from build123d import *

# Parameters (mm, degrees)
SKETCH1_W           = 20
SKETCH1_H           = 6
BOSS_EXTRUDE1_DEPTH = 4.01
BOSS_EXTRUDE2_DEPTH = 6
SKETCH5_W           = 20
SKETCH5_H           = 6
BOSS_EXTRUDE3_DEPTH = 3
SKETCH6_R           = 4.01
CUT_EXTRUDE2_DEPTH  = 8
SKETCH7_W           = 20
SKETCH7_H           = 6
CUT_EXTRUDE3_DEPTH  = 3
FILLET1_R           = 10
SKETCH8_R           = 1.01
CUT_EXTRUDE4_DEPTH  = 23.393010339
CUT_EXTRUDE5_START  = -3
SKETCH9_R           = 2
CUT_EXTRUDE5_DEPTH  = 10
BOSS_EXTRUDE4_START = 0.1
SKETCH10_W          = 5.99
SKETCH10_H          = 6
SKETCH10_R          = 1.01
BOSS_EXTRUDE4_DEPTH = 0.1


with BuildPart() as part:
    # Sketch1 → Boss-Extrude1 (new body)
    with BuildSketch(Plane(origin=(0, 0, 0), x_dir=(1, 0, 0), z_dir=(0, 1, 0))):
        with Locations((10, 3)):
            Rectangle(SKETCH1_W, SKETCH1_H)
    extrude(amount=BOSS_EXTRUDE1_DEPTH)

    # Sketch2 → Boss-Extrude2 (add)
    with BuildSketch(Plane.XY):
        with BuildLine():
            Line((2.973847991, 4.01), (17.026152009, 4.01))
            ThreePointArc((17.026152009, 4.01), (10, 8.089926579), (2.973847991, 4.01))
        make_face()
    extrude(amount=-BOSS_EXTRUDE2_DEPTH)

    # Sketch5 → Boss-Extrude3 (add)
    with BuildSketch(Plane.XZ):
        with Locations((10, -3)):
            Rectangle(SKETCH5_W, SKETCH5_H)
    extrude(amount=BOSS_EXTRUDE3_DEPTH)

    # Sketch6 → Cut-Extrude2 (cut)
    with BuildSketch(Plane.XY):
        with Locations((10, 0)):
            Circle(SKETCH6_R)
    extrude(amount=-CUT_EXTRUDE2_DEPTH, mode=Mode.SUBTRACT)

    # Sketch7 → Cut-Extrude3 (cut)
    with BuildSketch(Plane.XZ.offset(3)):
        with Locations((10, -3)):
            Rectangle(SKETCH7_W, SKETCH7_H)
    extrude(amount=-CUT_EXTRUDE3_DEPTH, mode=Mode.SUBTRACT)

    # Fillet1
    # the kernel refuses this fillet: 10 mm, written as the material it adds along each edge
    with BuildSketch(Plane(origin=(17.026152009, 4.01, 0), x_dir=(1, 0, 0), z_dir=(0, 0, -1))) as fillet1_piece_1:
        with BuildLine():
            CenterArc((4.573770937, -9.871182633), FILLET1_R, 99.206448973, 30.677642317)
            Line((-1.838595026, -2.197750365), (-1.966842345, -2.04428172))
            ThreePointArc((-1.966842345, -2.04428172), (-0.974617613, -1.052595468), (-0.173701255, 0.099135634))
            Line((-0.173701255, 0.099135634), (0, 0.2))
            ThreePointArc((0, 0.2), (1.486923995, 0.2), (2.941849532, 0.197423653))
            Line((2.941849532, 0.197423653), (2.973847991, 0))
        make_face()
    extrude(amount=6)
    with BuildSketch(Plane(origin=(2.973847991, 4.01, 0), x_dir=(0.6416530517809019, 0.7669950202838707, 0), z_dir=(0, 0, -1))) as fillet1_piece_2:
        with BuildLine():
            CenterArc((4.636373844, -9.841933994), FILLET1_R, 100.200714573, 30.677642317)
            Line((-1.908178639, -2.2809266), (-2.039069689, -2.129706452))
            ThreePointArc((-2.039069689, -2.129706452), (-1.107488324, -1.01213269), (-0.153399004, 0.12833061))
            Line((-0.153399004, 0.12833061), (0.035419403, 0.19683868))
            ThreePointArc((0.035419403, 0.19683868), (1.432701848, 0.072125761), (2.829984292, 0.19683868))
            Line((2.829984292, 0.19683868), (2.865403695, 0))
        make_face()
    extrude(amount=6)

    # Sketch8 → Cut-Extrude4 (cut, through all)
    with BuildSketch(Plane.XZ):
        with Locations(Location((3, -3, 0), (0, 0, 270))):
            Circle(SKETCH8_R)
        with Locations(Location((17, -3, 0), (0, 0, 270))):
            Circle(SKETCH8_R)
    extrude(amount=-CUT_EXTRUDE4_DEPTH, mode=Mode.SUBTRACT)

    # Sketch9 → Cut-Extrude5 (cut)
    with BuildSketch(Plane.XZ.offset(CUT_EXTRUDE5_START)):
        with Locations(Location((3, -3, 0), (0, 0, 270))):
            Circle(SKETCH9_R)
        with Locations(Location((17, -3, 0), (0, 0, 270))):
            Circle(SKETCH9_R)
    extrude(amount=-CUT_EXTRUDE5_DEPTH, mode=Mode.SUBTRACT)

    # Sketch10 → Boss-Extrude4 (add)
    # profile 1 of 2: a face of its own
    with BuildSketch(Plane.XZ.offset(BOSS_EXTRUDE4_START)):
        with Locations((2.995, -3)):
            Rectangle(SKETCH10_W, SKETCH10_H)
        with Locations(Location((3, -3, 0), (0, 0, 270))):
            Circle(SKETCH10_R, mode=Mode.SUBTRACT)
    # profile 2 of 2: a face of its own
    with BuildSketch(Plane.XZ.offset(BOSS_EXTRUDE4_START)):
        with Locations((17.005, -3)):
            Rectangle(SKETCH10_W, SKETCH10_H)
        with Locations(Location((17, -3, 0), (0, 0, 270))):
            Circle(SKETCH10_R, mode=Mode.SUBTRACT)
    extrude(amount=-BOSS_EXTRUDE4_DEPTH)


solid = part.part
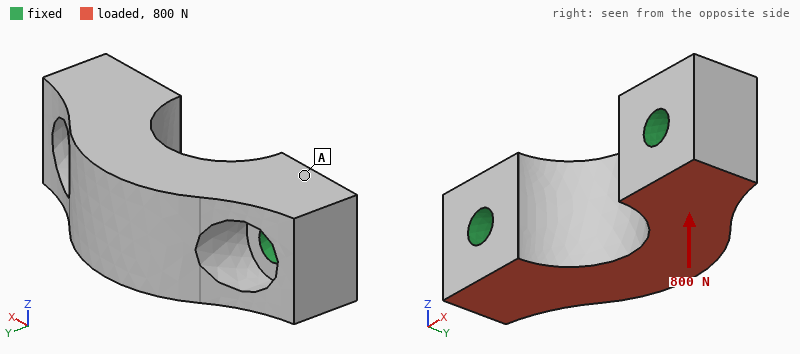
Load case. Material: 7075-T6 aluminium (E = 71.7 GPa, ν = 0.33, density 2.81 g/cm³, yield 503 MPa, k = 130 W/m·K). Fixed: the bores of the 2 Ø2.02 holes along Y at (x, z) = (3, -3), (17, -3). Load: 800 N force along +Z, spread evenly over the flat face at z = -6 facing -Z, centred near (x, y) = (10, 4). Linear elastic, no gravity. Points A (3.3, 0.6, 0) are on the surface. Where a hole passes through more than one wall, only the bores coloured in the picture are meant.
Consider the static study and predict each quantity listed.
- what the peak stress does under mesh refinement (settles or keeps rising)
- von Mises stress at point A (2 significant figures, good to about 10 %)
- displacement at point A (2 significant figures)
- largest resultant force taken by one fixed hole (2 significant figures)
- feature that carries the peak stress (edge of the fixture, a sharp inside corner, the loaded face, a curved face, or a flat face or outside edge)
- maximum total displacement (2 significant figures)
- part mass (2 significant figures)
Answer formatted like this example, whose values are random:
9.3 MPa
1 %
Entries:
keeps rising
20 MPa
2.0 µm
400 N
edge of the fixture
13 µm
1.5 g
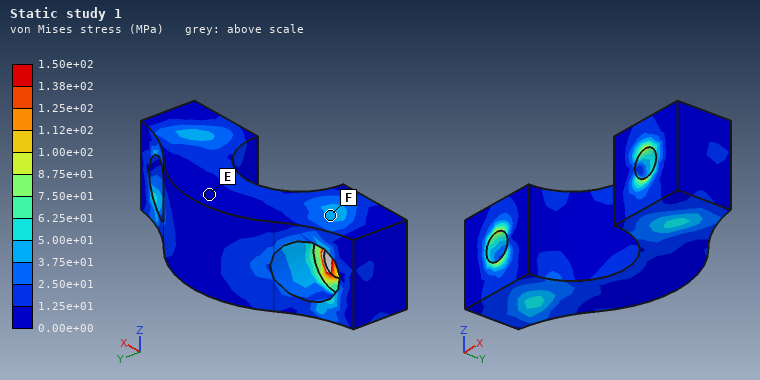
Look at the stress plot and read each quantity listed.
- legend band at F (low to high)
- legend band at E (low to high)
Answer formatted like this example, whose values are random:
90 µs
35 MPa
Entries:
3.75e+01 to 5.00e+01 MPa
0.00e+00 to 1.25e+01 MPa
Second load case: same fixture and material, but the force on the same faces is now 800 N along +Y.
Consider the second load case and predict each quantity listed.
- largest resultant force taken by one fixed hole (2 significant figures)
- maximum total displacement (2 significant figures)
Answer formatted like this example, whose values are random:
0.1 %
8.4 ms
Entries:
420 N
14 µm
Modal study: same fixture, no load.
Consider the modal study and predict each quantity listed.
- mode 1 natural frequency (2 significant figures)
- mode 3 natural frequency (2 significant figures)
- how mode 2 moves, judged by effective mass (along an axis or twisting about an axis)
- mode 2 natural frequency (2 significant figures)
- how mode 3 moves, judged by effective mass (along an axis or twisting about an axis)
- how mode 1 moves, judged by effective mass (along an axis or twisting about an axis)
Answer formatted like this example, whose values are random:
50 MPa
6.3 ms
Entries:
38 kHz
87 kHz
along Y
83 kHz
along X
along Z
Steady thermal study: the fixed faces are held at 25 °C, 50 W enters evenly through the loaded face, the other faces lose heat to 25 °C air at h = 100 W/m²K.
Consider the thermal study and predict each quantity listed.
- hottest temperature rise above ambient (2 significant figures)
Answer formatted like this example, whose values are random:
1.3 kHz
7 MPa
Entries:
38 K
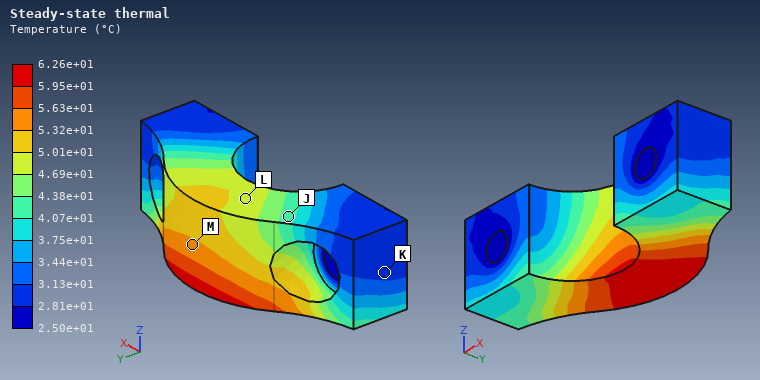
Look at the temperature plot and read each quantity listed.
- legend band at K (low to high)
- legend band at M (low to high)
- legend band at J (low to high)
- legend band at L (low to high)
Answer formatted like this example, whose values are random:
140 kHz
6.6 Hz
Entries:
2.81e+01 to 3.13e+01 °C
5.32e+01 to 5.63e+01 °C
4.07e+01 to 4.38e+01 °C
4.69e+01 to 5.01e+01 °C
